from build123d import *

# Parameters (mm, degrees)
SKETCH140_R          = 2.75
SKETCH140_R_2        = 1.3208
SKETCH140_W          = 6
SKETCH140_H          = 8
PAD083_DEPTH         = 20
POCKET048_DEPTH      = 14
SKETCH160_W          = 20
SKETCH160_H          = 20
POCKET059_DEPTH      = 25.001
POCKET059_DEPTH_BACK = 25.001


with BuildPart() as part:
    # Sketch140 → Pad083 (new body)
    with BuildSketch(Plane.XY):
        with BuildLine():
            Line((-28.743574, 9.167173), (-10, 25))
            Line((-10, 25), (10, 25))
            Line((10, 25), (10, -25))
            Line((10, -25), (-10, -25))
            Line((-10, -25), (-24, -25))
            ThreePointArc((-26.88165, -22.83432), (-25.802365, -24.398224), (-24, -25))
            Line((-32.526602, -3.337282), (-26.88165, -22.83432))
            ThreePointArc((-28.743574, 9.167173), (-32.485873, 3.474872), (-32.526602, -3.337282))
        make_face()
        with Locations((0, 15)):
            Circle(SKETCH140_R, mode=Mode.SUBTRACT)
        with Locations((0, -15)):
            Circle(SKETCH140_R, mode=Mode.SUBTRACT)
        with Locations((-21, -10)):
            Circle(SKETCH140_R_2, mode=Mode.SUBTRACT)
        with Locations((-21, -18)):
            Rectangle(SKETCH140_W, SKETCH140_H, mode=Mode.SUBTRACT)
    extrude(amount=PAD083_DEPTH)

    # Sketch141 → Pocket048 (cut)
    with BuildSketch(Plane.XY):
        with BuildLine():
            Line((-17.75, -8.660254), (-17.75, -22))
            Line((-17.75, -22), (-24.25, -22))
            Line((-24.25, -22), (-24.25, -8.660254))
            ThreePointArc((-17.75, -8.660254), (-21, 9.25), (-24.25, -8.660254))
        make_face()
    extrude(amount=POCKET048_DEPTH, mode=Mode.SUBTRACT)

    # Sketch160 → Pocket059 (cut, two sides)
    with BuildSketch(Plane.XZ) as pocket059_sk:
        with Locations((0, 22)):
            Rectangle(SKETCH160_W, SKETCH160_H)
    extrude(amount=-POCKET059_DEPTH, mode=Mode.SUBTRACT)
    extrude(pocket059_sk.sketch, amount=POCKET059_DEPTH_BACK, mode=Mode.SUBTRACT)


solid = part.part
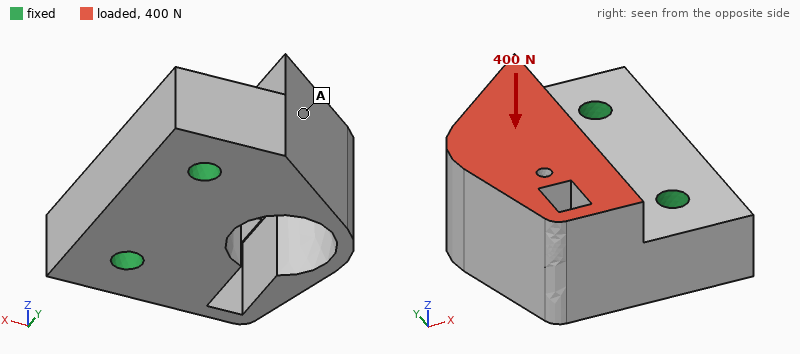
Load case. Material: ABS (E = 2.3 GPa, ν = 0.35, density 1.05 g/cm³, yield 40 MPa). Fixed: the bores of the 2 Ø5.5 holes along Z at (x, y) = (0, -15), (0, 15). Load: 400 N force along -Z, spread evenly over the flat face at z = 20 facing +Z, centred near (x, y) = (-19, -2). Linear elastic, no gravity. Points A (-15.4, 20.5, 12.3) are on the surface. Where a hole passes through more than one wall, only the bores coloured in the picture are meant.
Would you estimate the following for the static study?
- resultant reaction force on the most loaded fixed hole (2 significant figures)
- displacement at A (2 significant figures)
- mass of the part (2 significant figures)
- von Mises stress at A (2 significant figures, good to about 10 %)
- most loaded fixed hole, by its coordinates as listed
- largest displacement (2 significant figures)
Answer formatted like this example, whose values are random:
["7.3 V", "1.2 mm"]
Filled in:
["220 N", "0.072 mm", "24 g", "2.7 MPa", "(0, -15)", "0.25 mm"]
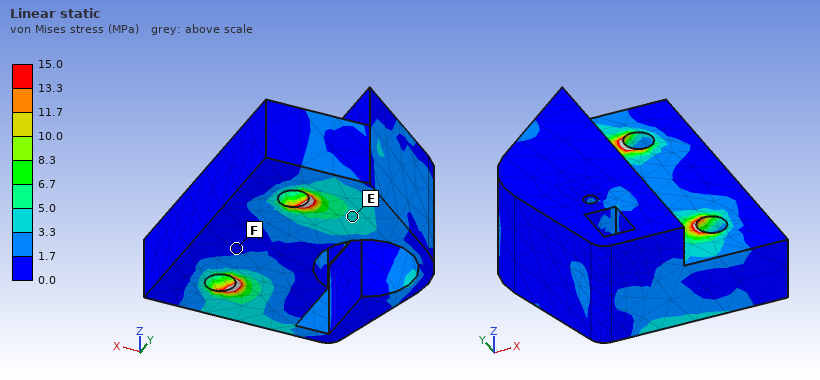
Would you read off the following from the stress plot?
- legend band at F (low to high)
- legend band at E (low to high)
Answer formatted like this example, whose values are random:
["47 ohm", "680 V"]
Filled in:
["0.0 to 1.7 MPa", "3.3 to 5.0 MPa"]
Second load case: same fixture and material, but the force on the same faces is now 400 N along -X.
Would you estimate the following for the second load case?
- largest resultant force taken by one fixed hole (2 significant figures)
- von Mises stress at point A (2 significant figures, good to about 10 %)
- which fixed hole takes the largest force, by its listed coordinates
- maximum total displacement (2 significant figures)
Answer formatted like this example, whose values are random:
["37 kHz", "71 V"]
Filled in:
["230 N", "3.8 MPa", "(0, -15)", "0.24 mm"]
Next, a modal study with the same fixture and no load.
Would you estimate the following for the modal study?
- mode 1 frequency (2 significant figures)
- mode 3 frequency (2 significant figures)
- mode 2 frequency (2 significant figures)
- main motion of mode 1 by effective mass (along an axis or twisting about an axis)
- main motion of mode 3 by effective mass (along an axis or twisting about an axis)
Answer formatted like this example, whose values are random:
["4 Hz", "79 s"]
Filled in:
["2300 Hz", "4900 Hz", "3800 Hz", "along Z", "along Y"]
